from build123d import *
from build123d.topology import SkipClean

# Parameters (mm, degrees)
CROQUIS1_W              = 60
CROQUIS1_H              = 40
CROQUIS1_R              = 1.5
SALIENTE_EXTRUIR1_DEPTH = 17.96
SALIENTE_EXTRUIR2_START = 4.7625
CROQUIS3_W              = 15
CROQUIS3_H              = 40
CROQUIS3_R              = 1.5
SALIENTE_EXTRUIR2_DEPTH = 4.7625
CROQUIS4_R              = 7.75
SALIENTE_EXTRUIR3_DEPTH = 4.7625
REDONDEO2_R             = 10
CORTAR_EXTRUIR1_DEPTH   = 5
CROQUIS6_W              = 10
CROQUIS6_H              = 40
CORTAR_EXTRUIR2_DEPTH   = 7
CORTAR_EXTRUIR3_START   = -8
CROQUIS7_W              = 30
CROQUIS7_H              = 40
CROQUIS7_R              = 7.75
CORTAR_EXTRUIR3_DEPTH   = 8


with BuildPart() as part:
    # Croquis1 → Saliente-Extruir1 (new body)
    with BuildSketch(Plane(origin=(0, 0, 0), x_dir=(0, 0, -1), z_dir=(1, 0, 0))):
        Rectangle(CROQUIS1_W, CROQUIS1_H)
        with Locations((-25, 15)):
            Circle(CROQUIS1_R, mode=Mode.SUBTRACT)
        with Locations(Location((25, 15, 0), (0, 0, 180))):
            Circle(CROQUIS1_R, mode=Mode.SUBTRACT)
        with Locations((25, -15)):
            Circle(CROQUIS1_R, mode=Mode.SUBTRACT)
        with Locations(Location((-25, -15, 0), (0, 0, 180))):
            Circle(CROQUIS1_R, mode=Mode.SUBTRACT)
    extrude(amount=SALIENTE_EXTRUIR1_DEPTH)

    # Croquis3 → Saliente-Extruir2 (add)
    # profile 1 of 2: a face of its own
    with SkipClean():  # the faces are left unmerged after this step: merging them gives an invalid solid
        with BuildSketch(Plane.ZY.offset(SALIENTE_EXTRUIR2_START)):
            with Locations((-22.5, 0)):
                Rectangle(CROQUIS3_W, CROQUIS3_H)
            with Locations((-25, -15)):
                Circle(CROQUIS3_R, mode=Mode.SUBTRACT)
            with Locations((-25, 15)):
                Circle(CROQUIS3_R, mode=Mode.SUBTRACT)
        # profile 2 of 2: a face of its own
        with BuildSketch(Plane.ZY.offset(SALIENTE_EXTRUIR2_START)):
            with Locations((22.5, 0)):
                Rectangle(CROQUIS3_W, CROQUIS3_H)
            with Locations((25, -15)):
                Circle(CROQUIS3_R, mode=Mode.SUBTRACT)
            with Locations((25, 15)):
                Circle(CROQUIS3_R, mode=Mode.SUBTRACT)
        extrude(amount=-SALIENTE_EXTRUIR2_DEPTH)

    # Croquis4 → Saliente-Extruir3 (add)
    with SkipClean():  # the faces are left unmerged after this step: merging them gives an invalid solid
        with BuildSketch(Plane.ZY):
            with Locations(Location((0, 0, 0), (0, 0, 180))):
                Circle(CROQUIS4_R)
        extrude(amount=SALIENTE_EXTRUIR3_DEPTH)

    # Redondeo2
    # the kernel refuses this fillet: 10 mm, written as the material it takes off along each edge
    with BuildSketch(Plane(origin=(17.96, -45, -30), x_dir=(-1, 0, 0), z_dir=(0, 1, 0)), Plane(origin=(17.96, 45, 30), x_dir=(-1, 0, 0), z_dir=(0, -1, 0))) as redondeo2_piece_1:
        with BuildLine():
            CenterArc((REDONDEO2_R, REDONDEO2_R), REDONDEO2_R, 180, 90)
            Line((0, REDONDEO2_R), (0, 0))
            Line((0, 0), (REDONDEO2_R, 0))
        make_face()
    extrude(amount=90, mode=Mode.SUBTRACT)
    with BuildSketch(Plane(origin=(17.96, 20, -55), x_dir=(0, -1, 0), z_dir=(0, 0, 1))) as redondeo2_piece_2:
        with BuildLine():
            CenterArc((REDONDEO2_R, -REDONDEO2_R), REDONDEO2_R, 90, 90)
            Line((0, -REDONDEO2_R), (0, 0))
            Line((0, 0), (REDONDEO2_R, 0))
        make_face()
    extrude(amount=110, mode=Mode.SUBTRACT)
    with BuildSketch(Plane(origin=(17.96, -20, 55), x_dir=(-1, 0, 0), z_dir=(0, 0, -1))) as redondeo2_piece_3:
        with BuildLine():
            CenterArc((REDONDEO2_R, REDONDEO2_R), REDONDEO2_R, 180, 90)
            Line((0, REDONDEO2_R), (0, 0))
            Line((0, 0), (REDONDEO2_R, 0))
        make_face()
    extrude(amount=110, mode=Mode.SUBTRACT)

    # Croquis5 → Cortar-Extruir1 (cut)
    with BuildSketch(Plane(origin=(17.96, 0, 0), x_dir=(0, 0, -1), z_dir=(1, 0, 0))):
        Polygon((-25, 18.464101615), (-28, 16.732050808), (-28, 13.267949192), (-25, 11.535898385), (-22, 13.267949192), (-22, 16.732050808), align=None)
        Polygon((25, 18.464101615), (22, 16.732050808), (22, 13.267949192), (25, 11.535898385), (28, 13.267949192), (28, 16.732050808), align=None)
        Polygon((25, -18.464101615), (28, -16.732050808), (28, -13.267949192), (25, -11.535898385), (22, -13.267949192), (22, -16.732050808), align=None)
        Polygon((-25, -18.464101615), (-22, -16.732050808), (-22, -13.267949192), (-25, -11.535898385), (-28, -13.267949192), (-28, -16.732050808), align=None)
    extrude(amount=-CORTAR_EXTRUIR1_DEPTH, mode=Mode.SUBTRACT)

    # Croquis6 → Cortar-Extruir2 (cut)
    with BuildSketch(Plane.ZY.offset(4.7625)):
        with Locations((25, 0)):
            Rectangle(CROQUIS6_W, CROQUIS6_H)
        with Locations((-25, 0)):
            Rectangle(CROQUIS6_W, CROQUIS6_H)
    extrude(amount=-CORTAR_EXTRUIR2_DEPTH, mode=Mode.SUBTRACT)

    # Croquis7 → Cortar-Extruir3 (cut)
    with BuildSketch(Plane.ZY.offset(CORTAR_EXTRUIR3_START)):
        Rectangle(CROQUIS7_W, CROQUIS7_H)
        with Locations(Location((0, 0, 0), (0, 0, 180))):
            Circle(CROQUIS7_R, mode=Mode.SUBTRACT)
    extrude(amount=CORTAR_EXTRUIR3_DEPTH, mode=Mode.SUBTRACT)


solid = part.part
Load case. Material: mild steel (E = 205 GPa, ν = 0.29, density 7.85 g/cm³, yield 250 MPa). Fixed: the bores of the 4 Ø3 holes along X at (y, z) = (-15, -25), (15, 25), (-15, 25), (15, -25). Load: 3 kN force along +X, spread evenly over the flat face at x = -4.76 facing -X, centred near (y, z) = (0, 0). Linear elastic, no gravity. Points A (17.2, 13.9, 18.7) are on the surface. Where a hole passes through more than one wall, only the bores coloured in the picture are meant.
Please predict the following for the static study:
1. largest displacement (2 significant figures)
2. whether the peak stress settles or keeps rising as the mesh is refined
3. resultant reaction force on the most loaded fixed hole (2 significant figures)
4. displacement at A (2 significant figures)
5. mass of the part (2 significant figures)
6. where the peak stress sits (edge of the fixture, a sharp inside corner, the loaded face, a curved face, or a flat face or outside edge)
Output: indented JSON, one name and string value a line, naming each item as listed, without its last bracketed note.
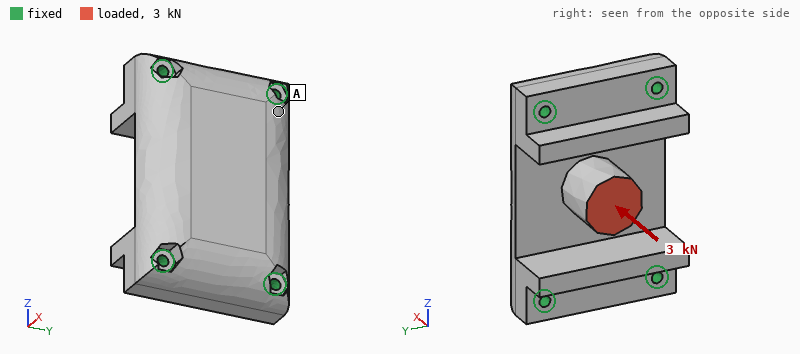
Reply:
{
  "largest displacement": "5.1 µm",
  "whether the peak stress settles or keeps rising as the mesh is refined": "keeps rising",
  "resultant reaction force on the most loaded fixed hole": "1.0 kN",
  "displacement at A": "1.4 µm",
  "mass of the part": "250 g",
  "where the peak stress sits": "edge of the fixture"
}
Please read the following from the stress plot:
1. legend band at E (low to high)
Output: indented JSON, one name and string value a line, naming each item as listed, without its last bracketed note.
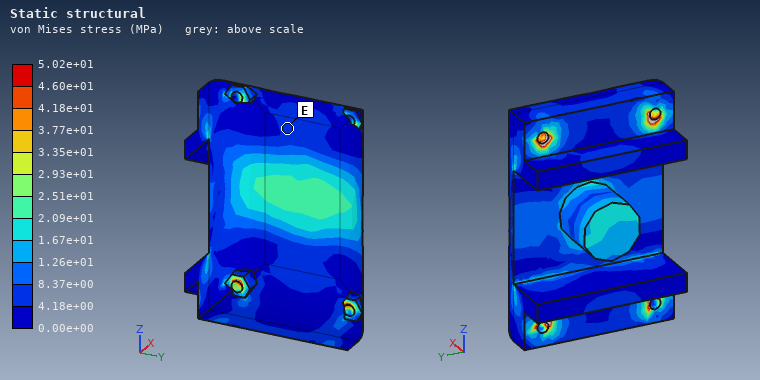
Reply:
{
  "legend band at E": "4.18e+00 to 8.37e+00 MPa"
}
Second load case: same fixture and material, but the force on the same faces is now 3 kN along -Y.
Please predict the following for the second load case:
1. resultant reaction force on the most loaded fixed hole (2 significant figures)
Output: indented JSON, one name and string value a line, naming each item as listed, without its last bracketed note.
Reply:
{
  "resultant reaction force on the most loaded fixed hole": "1000 N"
}
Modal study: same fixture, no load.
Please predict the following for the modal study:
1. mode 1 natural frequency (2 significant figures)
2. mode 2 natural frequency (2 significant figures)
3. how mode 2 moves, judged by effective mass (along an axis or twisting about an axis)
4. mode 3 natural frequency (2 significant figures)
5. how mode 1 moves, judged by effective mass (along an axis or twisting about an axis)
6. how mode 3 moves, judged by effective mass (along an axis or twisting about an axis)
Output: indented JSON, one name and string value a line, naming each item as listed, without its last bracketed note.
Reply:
{
  "mode 1 natural frequency": "14 kHz",
  "mode 2 natural frequency": "18 kHz",
  "how mode 2 moves, judged by effective mass": "along Y",
  "mode 3 natural frequency": "21 kHz",
  "how mode 1 moves, judged by effective mass": "along X",
  "how mode 3 moves, judged by effective mass": "along Z"
}
